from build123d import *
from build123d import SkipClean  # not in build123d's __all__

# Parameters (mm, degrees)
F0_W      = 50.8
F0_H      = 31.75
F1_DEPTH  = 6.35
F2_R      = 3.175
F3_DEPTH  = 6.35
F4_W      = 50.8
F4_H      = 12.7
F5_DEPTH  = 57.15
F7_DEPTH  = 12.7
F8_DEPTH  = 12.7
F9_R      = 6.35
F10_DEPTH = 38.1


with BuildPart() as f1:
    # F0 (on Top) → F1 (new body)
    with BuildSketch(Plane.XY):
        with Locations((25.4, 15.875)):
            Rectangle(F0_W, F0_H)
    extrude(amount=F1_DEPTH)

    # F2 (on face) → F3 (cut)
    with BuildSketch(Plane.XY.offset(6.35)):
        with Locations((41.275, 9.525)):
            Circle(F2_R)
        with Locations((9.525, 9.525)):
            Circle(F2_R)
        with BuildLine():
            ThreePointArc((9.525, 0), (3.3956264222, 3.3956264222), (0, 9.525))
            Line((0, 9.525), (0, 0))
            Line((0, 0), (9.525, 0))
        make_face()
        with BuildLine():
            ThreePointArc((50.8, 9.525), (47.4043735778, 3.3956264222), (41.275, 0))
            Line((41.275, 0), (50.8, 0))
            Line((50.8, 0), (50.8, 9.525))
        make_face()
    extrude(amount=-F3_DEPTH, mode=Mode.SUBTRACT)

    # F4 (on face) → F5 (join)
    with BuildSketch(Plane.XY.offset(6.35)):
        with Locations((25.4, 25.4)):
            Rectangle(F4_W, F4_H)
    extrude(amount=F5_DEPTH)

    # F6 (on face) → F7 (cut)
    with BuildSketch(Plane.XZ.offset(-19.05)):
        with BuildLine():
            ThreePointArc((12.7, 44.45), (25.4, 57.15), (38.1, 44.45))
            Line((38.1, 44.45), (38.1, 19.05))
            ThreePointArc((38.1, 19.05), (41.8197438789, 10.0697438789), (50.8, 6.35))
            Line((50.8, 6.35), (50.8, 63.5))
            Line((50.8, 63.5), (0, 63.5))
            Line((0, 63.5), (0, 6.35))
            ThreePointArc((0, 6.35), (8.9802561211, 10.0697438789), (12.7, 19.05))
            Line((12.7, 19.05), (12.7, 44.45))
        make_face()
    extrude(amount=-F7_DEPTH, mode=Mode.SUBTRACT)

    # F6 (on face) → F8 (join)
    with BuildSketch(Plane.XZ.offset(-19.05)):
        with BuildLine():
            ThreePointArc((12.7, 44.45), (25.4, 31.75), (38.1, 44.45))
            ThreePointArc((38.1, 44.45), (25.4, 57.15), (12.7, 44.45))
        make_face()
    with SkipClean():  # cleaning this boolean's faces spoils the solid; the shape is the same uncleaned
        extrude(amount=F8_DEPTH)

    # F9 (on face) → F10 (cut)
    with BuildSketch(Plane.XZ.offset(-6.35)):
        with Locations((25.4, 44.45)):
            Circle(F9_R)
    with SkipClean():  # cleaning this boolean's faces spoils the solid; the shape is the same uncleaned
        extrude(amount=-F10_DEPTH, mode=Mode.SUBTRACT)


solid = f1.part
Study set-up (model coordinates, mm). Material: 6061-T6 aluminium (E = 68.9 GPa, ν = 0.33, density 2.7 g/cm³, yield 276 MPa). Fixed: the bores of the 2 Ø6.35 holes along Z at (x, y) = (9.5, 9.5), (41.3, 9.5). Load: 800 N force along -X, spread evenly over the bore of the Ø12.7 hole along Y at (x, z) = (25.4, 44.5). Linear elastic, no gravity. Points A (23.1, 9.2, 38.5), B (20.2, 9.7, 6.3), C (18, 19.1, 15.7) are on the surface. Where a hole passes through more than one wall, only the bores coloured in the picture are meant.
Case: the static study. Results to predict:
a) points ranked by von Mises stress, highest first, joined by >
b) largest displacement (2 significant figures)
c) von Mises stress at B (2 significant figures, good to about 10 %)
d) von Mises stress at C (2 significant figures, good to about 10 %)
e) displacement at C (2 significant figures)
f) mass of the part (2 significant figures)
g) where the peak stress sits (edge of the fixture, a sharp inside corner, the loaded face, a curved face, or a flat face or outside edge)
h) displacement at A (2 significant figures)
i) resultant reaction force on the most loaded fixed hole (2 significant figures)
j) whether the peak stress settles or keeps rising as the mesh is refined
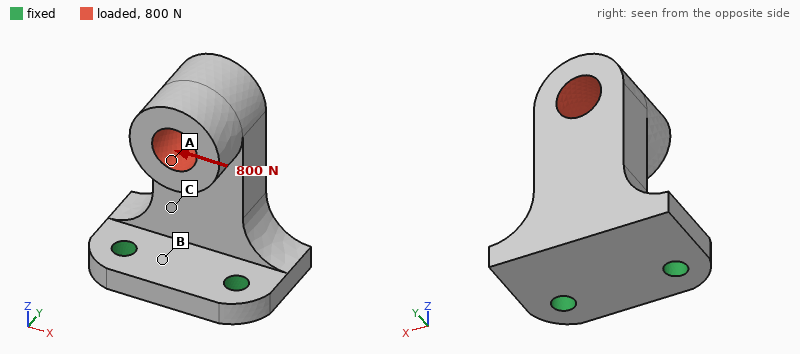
C > B > A
78 µm
11 MPa
19 MPa
15 µm
79 g
edge of the fixture
52 µm
1.1 kN
keeps rising
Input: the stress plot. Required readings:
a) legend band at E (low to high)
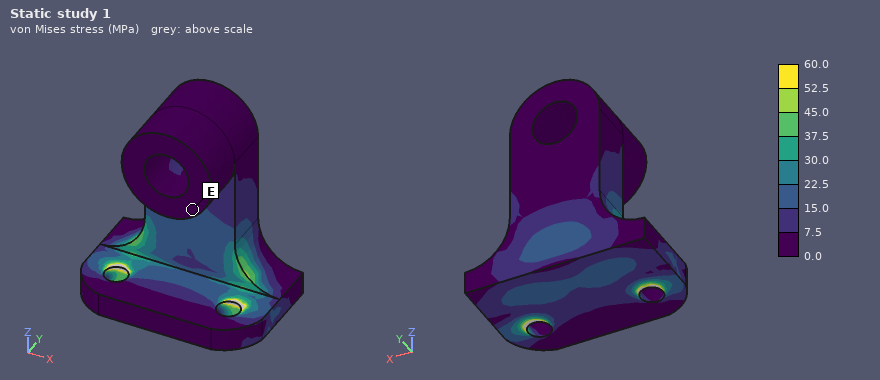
0.0 to 7.5 MPa
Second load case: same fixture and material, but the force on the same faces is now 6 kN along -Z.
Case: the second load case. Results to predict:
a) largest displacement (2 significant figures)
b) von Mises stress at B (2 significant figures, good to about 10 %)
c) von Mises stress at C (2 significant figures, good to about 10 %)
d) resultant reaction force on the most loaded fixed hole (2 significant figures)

0.10 mm
41 MPa
64 MPa
3.0 kN
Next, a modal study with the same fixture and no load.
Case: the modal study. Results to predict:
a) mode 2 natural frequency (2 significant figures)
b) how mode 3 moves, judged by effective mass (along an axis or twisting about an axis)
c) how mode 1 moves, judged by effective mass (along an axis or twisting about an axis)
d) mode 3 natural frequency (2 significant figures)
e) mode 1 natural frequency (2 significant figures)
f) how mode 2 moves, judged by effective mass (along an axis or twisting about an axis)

3400 Hz
along Z
along Y
6500 Hz
1500 Hz
along X
